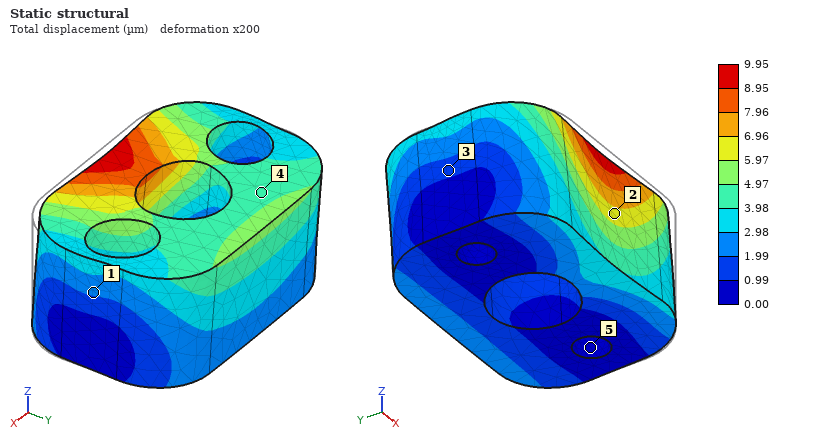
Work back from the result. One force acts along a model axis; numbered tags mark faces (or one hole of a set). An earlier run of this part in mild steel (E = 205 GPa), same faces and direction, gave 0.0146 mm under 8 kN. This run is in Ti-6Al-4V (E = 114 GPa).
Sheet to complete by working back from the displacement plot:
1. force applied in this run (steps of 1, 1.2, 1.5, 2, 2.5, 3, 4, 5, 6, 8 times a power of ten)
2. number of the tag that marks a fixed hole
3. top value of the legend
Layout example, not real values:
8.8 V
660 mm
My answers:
3 kN
5
9.95 µm
